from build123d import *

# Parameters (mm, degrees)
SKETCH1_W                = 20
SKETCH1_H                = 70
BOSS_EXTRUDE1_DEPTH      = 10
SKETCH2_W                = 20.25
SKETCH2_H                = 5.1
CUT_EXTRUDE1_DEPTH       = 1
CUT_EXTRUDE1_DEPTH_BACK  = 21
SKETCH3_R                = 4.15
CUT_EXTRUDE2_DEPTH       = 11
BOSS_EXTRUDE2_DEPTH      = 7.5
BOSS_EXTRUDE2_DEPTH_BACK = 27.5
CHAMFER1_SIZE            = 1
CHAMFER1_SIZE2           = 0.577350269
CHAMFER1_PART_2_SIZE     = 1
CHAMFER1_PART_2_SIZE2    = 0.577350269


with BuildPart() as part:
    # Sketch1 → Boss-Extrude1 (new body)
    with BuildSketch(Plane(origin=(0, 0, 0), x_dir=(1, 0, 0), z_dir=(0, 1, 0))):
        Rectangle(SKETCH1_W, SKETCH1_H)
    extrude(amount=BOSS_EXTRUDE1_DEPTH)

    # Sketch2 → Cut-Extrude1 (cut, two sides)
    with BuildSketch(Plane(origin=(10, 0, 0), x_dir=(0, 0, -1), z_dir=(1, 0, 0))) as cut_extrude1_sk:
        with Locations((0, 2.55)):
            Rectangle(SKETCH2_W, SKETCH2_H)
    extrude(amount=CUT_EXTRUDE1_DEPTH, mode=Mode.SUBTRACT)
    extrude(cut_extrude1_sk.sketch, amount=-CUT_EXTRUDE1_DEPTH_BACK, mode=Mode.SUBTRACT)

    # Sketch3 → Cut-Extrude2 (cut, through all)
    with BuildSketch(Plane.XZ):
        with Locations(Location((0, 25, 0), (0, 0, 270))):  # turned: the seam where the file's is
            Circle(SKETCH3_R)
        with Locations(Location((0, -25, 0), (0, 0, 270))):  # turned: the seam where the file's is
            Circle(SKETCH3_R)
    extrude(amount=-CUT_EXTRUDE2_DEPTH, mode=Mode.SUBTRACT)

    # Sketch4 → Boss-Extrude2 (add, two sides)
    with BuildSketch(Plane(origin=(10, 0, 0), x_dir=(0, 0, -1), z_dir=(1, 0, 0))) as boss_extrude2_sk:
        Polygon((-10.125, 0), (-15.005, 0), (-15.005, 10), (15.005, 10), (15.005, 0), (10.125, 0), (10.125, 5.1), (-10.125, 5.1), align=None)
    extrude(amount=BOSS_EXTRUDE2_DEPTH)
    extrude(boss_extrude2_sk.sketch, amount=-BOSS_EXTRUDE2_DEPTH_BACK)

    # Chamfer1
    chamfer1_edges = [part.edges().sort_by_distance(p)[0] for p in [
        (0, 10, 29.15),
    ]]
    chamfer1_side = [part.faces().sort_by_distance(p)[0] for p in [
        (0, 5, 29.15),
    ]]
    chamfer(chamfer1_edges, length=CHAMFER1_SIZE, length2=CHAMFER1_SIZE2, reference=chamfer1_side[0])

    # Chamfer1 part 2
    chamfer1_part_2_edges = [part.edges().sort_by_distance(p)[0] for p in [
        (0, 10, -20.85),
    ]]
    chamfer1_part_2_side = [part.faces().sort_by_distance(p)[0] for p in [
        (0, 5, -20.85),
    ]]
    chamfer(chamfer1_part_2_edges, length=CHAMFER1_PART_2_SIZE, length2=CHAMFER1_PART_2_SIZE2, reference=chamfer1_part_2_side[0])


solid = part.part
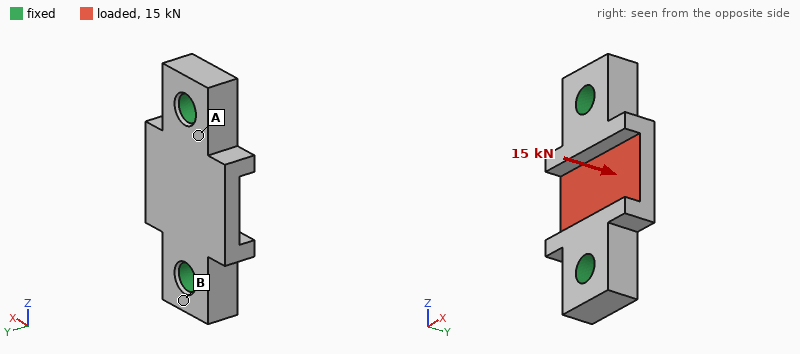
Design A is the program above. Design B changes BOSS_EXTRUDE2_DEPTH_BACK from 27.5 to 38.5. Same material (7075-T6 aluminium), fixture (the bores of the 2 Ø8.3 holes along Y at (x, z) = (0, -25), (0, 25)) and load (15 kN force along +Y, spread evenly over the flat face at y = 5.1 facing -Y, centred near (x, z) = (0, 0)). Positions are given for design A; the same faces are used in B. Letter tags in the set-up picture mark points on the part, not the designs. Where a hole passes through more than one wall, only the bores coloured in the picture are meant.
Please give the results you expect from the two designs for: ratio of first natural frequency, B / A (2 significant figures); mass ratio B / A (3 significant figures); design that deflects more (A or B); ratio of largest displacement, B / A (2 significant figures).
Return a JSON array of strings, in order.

["0.52", "1.16", "B", "2.6"]
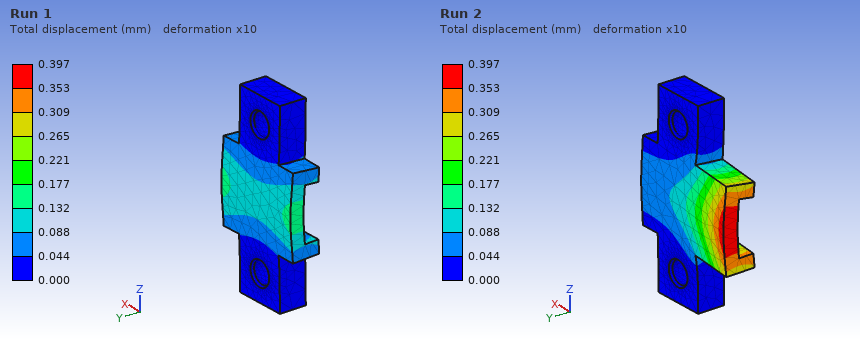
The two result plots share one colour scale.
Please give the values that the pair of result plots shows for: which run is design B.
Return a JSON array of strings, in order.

["Run 2"]
